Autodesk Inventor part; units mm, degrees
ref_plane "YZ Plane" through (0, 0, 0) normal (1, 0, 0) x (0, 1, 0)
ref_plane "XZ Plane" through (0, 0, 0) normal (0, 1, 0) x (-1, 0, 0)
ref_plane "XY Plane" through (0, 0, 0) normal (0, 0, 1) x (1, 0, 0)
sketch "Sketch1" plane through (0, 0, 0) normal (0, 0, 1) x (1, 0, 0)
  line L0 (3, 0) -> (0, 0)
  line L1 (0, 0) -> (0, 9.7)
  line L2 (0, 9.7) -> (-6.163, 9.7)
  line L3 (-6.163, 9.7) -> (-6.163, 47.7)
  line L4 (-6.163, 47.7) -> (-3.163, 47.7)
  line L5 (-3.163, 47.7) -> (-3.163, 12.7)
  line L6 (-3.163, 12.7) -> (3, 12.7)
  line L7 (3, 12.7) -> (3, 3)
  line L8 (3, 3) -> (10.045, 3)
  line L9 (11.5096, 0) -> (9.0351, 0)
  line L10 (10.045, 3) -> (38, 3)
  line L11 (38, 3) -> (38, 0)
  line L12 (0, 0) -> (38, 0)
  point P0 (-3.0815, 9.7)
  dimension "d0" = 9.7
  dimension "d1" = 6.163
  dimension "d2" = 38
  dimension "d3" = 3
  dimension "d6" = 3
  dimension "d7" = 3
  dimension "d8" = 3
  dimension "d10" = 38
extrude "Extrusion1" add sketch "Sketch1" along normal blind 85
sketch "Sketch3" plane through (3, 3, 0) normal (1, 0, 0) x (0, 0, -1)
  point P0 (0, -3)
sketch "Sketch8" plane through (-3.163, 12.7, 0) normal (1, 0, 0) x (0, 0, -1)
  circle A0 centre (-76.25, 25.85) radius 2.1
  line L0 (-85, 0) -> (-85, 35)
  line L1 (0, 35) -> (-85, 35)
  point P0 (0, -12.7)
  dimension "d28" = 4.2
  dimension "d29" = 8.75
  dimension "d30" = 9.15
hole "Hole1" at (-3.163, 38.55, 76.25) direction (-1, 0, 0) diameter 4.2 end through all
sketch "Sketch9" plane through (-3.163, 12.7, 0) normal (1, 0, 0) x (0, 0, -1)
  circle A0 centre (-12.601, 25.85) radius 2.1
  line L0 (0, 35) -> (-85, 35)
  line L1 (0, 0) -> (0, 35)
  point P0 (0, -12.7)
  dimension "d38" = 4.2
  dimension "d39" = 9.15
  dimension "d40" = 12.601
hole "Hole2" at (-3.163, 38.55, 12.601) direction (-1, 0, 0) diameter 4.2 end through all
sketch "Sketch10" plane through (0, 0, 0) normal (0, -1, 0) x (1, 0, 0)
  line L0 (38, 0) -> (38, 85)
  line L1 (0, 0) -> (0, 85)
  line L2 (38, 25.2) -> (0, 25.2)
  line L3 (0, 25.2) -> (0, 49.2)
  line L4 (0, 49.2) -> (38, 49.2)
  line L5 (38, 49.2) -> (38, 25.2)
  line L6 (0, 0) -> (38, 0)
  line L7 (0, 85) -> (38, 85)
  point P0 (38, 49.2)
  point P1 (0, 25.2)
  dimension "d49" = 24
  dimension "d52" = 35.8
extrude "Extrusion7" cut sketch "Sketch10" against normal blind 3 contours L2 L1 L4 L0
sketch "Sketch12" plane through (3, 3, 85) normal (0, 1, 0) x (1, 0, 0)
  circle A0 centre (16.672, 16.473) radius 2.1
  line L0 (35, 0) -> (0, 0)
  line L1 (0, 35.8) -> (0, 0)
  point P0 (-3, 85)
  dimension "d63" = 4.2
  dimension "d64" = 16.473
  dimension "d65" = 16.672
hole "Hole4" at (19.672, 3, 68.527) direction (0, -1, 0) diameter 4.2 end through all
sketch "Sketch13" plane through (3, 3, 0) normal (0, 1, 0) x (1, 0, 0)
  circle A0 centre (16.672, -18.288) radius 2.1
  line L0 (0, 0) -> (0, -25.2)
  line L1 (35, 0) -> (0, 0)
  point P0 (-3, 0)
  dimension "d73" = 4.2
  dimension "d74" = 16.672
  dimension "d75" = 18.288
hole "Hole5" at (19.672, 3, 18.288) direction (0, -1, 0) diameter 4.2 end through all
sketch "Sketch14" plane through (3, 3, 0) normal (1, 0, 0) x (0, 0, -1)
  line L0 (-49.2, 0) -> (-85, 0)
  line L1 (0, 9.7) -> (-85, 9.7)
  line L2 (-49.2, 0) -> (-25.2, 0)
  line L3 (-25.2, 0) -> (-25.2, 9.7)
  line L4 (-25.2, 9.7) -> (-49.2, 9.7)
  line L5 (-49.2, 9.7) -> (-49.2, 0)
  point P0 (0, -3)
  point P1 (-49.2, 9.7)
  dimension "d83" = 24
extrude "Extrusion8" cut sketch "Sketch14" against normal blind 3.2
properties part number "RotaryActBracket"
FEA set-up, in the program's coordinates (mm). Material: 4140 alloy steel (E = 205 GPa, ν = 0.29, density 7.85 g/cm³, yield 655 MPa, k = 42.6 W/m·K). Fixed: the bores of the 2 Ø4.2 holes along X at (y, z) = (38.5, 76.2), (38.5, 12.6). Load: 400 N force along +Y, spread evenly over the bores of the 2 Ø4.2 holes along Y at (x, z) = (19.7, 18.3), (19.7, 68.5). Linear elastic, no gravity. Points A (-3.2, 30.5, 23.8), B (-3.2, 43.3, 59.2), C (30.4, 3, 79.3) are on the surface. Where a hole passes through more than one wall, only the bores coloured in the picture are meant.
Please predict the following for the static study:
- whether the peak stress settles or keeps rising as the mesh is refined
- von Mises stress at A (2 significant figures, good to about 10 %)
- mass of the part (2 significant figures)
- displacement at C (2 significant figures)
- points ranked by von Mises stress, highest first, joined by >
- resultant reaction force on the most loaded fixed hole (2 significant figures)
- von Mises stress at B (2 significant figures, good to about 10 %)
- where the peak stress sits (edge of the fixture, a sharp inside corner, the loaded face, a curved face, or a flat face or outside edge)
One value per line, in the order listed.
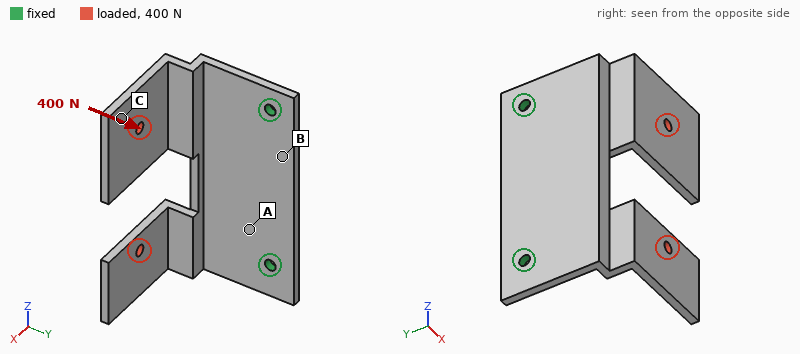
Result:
keeps rising
73 MPa
150 g
0.45 mm
A > B > C
210 N
41 MPa
edge of the fixture
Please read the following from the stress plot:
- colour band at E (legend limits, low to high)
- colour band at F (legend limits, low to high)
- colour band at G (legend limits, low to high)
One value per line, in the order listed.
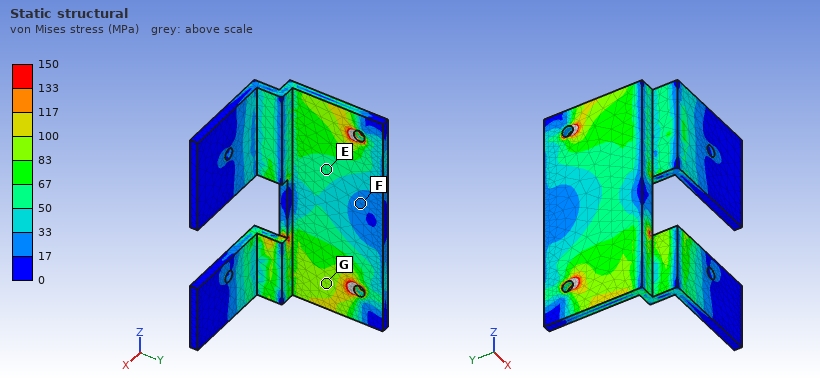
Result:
50 to 67 MPa
17 to 33 MPa
83 to 100 MPa
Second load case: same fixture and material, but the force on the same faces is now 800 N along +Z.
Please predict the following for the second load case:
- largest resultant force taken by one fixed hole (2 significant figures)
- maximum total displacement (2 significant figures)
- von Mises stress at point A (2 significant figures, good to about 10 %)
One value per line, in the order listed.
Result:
670 N
0.36 mm
57 MPa
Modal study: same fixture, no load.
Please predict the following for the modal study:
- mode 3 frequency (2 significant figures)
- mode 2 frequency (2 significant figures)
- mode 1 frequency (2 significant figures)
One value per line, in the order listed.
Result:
1400 Hz
720 Hz
550 Hz
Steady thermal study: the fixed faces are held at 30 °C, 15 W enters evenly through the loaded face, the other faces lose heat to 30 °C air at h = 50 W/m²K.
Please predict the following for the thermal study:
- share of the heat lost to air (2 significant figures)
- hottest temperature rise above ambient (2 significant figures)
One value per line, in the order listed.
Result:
81 %
60 K
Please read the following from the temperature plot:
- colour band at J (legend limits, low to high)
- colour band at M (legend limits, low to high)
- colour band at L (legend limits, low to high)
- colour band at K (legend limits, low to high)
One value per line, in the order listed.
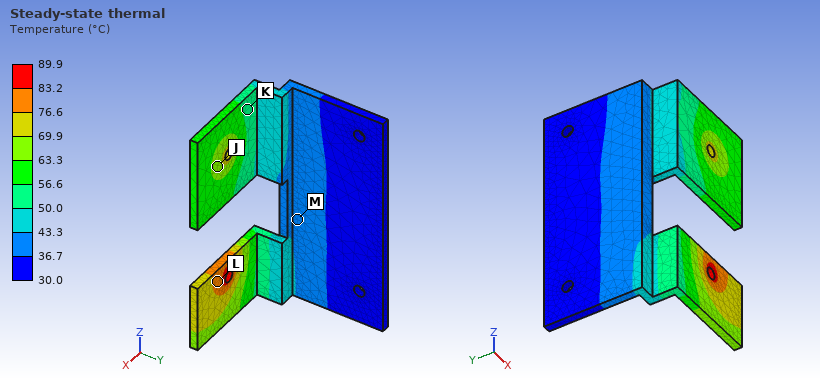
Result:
63.3 to 69.9 °C
36.7 to 43.3 °C
76.6 to 83.2 °C
50.0 to 56.6 °C
